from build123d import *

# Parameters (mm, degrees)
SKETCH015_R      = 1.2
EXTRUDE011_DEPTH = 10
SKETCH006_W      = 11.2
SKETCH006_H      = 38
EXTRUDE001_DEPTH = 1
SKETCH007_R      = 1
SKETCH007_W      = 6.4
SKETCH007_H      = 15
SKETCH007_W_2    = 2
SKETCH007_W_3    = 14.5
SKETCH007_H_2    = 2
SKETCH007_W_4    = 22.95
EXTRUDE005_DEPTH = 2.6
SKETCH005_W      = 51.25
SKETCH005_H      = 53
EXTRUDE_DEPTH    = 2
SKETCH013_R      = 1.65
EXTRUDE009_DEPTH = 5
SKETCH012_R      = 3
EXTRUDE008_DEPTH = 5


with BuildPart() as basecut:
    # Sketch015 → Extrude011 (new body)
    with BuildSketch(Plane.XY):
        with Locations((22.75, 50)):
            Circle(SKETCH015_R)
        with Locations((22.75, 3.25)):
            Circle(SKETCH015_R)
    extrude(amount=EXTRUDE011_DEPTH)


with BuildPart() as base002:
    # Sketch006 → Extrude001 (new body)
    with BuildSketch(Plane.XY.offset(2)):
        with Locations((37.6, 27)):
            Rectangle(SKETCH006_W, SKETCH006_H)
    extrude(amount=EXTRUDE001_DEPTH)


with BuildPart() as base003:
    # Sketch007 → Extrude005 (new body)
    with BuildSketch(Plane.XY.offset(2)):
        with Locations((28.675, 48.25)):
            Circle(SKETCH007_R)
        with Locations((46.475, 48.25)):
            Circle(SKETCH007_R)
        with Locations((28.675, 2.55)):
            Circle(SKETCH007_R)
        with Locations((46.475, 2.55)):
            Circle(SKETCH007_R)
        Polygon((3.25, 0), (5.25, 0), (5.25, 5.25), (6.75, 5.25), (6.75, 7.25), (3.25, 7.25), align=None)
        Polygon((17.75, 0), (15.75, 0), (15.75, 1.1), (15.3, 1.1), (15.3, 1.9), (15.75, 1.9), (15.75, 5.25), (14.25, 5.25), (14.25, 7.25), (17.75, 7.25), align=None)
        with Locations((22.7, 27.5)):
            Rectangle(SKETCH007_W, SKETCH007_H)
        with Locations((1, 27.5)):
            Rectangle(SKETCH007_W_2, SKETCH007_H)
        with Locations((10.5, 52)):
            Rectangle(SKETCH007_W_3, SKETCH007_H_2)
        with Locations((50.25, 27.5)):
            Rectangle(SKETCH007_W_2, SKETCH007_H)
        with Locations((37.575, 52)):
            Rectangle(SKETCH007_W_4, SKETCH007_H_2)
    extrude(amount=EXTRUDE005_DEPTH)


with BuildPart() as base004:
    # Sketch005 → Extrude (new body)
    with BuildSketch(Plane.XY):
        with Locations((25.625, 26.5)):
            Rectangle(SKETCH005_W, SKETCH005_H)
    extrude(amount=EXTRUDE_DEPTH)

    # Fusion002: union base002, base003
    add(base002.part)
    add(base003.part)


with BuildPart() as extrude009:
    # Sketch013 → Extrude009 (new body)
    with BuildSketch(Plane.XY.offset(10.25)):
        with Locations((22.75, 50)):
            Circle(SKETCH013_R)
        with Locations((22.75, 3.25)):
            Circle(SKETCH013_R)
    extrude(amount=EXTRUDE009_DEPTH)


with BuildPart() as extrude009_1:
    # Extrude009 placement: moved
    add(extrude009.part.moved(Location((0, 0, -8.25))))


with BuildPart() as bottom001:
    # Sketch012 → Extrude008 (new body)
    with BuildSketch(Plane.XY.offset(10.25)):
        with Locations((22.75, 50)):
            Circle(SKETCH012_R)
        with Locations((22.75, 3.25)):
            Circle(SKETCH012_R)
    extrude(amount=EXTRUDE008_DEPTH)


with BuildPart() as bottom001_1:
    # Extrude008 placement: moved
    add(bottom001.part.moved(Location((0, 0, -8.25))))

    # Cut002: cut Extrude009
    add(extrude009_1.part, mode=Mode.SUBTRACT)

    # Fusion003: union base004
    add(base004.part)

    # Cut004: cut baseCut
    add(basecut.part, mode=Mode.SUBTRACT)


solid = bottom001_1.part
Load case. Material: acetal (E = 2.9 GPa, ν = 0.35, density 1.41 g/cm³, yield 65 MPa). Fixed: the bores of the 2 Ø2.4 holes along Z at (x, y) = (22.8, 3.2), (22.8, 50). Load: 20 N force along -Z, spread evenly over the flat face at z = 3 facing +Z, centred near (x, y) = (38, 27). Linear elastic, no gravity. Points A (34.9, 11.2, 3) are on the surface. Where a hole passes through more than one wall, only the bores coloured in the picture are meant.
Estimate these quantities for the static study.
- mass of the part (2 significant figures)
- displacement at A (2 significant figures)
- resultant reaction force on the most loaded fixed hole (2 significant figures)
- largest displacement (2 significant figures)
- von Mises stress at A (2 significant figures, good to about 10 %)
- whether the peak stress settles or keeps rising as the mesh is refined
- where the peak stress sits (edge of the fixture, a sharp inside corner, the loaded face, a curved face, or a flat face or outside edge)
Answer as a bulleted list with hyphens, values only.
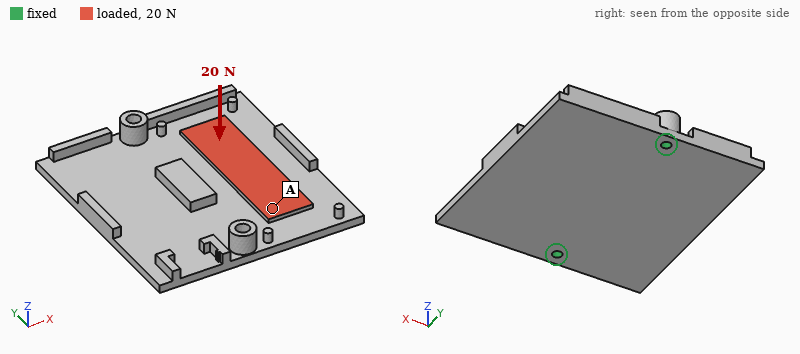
- 9.5 g
- 0.29 mm
- 12 N
- 0.81 mm
- 2.3 MPa
- keeps rising
- edge of the fixture
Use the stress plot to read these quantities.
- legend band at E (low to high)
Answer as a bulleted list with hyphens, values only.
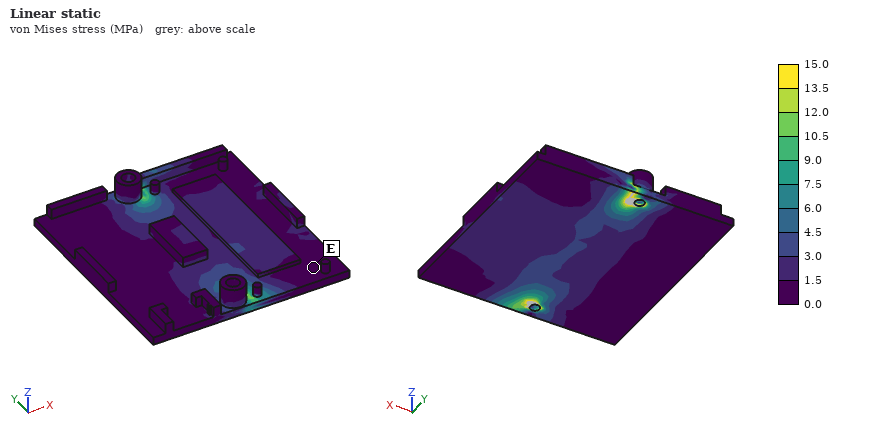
- 0.0 to 1.5 MPa
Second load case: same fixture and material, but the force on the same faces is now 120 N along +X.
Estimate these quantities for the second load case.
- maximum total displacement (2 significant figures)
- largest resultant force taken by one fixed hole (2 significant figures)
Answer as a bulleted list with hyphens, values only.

- 0.76 mm
- 61 N
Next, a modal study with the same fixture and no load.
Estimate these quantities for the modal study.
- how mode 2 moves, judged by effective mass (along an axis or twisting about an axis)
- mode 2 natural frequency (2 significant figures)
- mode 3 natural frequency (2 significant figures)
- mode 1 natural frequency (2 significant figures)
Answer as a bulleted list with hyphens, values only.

- along Z
- 730 Hz
- 1100 Hz
- 420 Hz
